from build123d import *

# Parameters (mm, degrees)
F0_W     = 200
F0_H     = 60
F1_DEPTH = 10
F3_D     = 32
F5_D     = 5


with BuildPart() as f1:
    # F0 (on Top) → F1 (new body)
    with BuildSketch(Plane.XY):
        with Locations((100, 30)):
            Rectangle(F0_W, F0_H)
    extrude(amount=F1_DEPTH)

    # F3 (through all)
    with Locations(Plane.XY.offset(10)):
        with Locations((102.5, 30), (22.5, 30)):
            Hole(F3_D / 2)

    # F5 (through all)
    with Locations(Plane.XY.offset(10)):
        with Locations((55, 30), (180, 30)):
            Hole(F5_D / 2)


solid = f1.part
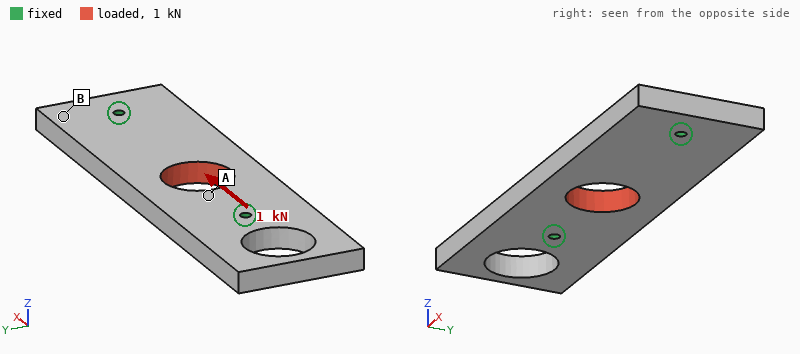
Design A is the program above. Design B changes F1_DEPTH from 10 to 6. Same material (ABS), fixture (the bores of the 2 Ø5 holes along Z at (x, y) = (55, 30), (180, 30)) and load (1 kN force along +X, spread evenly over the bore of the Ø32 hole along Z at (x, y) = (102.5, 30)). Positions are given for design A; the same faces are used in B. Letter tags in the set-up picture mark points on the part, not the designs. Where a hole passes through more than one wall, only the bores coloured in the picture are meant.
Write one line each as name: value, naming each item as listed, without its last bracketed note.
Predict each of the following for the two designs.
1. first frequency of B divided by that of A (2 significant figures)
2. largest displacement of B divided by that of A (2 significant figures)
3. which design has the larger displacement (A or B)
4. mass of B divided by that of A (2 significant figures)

first frequency of B divided by that of A: 0.65
largest displacement of B divided by that of A: 1.7
which design has the larger displacement: B
mass of B divided by that of A: 0.60
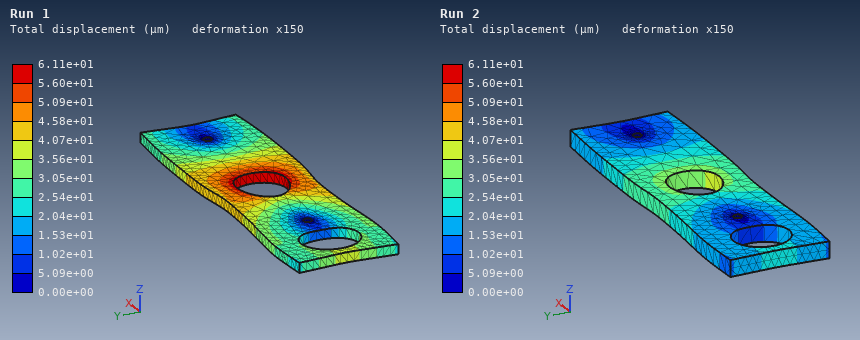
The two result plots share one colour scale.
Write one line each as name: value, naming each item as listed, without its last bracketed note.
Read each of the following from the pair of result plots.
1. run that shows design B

run that shows design B: Run 1
